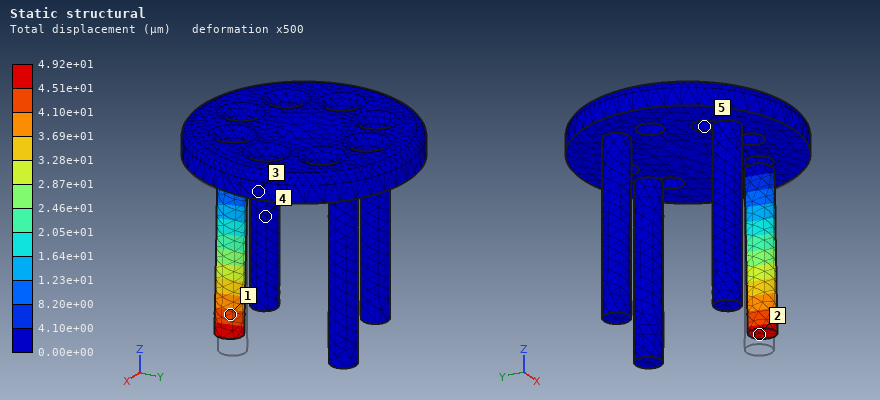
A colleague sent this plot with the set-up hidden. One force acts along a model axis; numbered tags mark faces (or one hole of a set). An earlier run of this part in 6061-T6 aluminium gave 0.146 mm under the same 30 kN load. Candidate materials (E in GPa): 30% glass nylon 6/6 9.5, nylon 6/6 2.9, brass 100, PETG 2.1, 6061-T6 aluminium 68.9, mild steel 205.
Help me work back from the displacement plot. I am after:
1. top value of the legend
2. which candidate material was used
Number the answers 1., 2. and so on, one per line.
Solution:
1. 4.92e+01 µm
2. mild steel
